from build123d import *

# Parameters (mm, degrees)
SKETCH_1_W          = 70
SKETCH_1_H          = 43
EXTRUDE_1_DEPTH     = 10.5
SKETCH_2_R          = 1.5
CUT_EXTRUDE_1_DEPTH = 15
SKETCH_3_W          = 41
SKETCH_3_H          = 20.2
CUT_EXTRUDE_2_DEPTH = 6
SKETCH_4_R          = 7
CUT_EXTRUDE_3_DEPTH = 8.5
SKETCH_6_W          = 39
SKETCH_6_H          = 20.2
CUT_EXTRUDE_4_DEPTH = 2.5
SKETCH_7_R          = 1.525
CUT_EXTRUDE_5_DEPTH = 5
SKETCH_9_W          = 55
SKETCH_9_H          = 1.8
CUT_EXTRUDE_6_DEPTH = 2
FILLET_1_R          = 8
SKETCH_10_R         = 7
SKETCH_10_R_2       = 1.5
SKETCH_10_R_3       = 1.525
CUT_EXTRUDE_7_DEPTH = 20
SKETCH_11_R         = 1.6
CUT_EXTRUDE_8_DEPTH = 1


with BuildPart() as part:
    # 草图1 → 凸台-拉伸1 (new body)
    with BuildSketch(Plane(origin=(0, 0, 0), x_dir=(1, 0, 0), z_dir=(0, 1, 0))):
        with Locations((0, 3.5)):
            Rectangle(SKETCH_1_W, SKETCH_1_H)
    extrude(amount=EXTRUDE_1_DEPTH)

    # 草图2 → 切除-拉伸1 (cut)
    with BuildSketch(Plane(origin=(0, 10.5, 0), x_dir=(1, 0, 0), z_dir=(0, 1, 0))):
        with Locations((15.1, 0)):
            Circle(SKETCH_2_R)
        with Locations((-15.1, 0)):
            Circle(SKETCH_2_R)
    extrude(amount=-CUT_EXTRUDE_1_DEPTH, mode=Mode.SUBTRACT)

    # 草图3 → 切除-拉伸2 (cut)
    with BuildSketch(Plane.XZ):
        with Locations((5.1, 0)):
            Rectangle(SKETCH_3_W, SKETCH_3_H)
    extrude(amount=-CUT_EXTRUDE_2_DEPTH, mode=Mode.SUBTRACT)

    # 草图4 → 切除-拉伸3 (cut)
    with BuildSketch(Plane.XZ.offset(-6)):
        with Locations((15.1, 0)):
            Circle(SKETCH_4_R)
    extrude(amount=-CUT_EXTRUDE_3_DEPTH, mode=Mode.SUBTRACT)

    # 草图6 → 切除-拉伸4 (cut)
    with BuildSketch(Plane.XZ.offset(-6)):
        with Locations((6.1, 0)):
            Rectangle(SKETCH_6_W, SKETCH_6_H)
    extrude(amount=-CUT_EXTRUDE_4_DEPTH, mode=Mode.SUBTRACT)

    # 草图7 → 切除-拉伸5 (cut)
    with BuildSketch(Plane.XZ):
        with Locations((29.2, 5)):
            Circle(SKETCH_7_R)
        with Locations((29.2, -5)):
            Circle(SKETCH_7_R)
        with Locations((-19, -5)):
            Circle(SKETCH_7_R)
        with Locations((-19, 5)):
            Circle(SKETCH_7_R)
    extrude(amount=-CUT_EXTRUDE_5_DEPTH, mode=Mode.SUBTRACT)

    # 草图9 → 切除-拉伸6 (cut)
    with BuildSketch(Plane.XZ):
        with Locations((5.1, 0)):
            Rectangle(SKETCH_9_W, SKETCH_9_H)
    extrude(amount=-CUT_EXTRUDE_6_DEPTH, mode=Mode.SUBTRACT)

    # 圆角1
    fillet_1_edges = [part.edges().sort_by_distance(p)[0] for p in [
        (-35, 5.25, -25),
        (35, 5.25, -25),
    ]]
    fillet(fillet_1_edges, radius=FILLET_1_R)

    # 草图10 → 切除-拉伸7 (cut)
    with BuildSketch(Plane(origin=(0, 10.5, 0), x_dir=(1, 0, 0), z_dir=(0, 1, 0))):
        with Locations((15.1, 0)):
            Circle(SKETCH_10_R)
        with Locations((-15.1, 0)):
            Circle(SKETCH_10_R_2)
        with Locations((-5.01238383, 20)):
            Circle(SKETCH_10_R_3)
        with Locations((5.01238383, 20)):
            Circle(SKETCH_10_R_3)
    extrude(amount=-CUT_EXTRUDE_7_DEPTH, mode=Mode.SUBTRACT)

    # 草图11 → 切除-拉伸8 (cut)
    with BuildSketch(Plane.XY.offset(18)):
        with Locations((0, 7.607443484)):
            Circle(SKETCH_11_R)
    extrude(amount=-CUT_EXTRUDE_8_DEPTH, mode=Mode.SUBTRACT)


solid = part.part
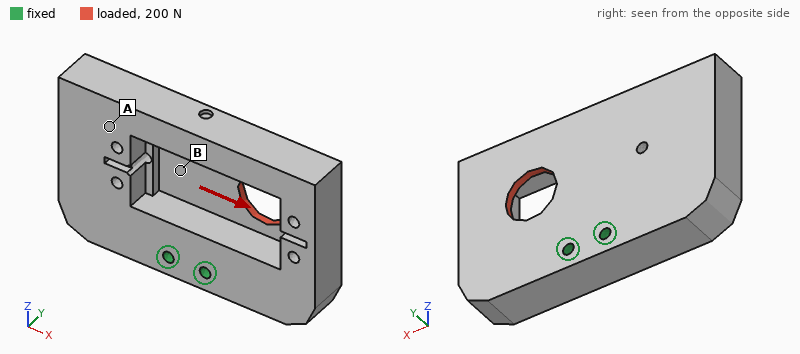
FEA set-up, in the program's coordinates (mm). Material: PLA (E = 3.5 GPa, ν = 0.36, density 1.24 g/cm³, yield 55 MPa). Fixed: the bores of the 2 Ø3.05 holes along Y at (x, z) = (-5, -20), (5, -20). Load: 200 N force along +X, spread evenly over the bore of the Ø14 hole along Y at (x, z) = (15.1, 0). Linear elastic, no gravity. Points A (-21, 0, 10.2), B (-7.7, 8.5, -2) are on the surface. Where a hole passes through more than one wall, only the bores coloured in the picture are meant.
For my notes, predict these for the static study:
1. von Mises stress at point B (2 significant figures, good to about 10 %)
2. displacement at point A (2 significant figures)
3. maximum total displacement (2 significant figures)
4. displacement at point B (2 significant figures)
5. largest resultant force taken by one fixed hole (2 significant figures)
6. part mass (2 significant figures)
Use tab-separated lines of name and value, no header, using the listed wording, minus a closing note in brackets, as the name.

von Mises stress at point B	2.5 MPa
displacement at point A	0.091 mm
maximum total displacement	0.14 mm
displacement at point B	0.050 mm
largest resultant force taken by one fixed hole	310 N
part mass	29 g
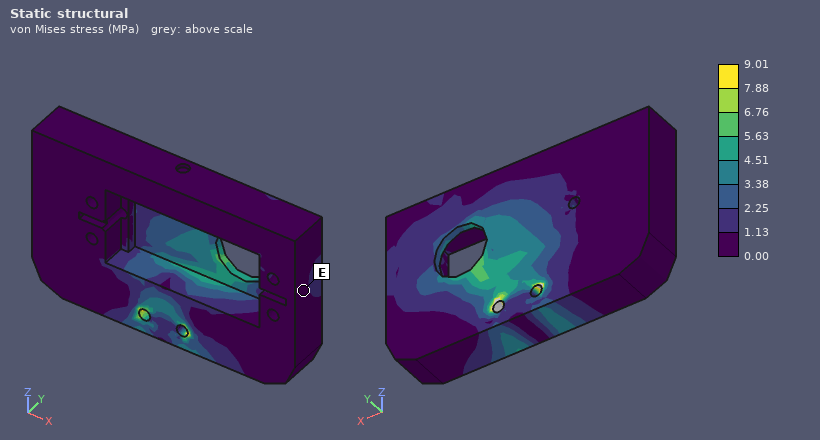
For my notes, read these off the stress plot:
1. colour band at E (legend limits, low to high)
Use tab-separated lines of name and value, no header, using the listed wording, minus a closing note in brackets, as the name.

colour band at E	0.00 to 1.13 MPa
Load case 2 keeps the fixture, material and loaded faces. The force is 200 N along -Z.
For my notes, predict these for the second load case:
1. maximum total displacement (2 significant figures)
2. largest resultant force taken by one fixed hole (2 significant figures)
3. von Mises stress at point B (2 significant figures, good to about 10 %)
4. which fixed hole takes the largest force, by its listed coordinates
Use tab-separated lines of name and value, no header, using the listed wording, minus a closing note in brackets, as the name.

maximum total displacement	0.11 mm
largest resultant force taken by one fixed hole	320 N
von Mises stress at point B	1.1 MPa
which fixed hole takes the largest force, by its listed coordinates	(5, -20)
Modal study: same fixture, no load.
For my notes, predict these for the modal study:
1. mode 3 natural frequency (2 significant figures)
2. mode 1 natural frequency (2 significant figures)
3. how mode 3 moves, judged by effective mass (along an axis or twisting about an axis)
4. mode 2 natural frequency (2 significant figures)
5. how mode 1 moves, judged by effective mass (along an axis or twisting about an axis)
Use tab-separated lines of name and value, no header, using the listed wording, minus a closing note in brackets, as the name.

mode 3 natural frequency	1300 Hz
mode 1 natural frequency	900 Hz
how mode 3 moves, judged by effective mass	along X
mode 2 natural frequency	1100 Hz
how mode 1 moves, judged by effective mass	along Y
